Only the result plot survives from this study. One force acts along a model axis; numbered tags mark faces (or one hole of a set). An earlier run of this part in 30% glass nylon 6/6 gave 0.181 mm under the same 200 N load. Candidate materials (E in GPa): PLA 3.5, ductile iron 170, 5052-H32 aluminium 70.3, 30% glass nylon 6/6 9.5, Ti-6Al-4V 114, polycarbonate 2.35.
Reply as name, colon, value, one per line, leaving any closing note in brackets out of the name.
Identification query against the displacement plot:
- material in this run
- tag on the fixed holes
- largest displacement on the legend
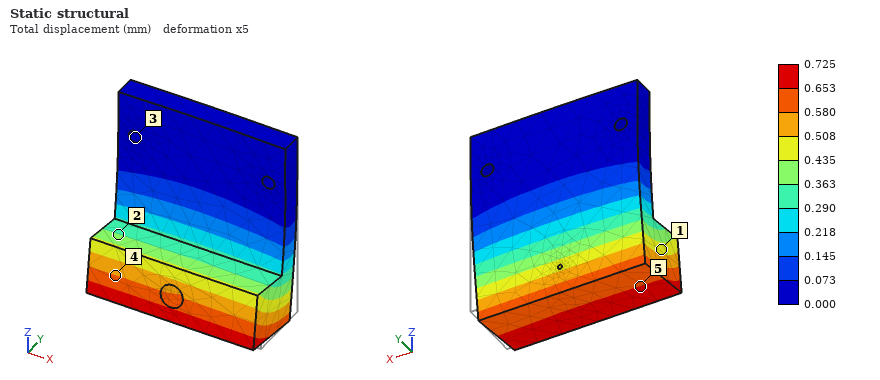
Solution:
material in this run: polycarbonate
tag on the fixed holes: 3
largest displacement on the legend: 0.725 mm
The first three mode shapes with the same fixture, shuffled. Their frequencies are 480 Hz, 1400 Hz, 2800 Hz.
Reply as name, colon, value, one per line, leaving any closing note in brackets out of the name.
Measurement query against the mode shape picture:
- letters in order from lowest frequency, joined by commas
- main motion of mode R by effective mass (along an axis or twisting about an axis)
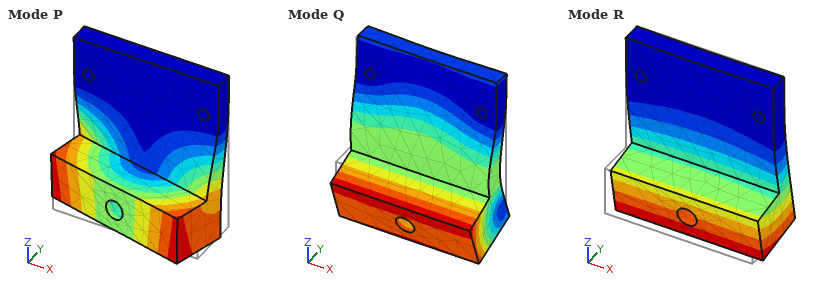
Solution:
letters in order from lowest frequency, joined by commas: R, P, Q
main motion of mode R by effective mass: along Y
